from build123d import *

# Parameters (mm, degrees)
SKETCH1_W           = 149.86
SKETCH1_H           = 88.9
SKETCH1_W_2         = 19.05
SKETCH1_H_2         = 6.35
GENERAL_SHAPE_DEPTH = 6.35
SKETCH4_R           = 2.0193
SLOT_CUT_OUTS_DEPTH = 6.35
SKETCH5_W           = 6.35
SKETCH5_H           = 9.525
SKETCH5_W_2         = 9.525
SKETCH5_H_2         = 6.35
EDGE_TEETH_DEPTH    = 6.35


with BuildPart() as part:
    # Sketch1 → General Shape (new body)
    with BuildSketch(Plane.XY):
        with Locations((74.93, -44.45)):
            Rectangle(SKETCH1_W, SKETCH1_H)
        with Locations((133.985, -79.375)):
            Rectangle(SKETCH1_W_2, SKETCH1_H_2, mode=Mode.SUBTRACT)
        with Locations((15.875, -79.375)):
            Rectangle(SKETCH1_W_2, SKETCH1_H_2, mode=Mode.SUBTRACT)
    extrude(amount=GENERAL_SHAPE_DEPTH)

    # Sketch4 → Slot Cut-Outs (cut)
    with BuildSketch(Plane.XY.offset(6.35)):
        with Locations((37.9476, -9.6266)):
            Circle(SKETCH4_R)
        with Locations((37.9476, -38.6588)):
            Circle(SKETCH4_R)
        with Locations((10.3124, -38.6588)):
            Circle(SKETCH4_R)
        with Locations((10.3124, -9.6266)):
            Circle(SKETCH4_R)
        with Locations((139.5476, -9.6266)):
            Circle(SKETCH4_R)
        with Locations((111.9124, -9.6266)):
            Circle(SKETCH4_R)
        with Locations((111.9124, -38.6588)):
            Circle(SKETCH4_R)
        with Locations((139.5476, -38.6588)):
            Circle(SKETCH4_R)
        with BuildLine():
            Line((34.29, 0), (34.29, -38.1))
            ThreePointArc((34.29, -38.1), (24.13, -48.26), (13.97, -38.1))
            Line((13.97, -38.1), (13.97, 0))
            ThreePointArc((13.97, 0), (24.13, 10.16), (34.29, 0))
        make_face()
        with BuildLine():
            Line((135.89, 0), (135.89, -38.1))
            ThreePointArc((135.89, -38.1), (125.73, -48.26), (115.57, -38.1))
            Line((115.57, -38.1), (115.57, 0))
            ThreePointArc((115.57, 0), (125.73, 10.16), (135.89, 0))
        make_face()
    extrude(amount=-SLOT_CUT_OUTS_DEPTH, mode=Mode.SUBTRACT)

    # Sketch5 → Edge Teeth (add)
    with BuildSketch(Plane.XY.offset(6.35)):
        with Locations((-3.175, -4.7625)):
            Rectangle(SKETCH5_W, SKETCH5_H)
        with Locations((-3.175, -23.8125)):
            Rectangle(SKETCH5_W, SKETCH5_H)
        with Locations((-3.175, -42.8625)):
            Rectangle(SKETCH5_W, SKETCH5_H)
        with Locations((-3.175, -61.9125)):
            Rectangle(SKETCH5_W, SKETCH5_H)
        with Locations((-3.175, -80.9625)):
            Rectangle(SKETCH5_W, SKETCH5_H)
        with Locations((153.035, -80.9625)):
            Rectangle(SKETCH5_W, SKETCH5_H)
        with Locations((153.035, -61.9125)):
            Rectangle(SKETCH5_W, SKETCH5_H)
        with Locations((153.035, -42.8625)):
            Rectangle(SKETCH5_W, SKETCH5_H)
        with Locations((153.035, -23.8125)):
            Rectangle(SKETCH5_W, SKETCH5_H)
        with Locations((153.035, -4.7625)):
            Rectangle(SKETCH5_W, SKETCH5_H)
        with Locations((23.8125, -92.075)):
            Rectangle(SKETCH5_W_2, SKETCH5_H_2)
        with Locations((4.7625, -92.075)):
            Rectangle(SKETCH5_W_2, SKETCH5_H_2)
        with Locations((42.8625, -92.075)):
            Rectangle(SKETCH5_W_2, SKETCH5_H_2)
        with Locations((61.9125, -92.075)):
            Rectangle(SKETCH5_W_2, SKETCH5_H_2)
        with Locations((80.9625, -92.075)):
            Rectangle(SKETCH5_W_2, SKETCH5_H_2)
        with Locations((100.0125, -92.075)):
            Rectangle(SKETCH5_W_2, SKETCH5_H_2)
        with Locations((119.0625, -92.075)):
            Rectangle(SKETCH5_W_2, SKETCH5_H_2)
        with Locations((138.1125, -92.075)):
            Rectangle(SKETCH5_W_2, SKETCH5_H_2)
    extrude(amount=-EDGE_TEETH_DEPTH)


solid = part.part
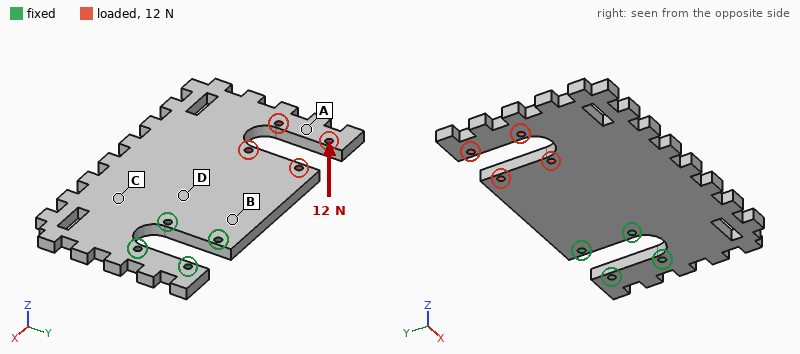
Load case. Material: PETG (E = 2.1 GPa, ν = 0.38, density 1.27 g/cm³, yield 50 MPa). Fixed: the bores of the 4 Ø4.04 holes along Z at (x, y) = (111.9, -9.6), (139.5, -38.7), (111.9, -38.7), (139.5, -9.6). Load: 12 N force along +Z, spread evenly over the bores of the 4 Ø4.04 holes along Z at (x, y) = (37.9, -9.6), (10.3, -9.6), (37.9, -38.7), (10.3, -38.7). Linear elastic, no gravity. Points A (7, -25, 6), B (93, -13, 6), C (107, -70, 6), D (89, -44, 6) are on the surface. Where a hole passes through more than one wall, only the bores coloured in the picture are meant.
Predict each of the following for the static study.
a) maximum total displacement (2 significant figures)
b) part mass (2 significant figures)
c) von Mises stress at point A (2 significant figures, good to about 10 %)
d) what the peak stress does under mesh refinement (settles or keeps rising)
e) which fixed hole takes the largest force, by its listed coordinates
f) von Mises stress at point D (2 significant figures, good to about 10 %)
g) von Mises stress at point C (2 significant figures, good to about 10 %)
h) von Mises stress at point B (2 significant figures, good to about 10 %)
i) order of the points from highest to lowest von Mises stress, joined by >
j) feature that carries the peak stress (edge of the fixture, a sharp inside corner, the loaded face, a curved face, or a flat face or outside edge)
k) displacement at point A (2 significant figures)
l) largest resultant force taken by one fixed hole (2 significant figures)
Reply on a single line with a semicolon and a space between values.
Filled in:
1.8 mm; 98 g; 0.48 MPa; keeps rising; (111.9, -38.7); 1.2 MPa; 0.97 MPa; 1.5 MPa; B > D > C > A; edge of the fixture; 1.3 mm; 18 N
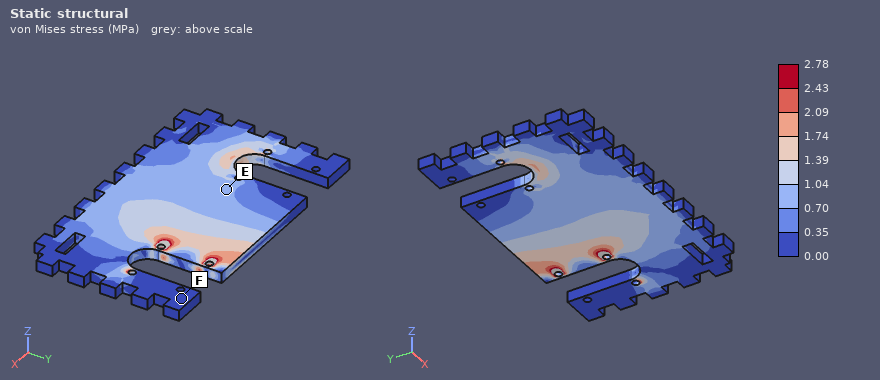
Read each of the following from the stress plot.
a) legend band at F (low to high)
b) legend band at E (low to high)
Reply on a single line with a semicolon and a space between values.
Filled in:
0.00 to 0.35 MPa; 0.70 to 1.04 MPa
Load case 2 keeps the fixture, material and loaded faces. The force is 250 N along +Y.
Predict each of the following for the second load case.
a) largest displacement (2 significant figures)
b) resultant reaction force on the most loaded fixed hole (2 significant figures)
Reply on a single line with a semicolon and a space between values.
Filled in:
0.52 mm; 490 N
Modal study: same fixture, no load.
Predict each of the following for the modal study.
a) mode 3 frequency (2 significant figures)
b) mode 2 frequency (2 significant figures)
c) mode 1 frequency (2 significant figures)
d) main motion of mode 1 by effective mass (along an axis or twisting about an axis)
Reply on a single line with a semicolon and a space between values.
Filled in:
400 Hz; 200 Hz; 94 Hz; along Z
